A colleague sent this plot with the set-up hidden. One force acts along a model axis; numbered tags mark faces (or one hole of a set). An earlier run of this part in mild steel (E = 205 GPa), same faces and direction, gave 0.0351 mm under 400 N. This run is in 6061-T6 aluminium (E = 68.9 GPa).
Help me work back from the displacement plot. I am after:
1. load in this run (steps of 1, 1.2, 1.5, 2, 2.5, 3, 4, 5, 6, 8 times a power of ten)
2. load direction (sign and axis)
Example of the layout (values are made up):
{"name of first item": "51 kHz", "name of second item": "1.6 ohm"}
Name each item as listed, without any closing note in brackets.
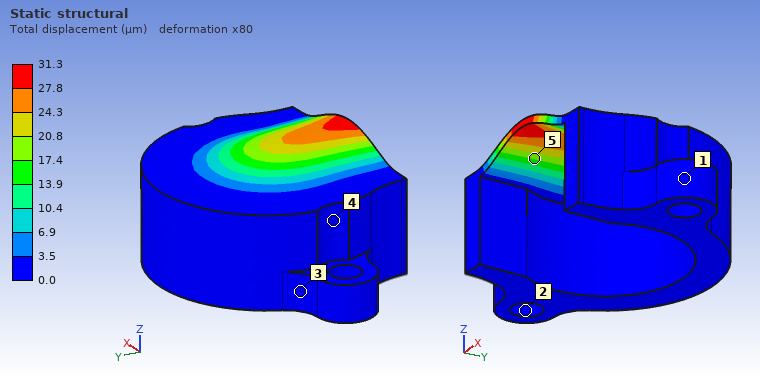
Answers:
{"load in this run": "120 N", "load direction": "+Z"}
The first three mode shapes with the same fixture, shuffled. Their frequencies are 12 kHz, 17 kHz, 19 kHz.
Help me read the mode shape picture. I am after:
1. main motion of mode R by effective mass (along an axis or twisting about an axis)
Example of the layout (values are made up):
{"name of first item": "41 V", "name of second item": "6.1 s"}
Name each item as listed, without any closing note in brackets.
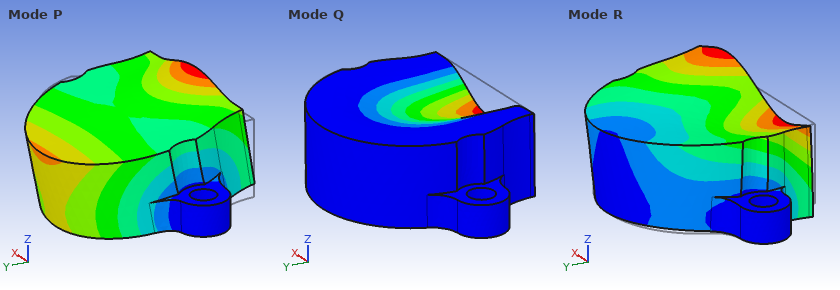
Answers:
{"main motion of mode R by effective mass": "along X"}
